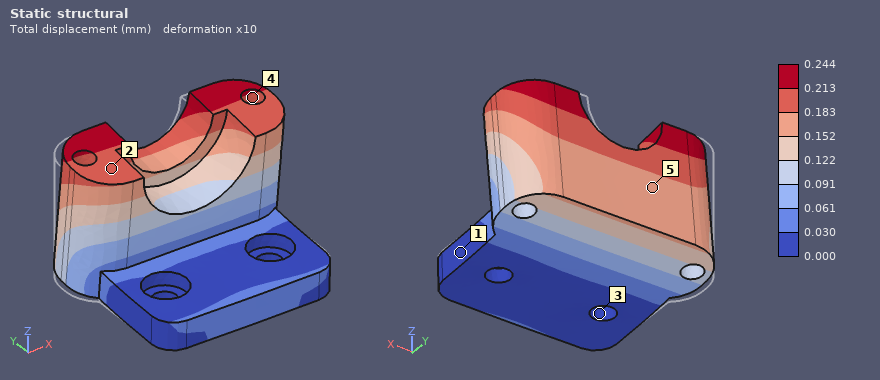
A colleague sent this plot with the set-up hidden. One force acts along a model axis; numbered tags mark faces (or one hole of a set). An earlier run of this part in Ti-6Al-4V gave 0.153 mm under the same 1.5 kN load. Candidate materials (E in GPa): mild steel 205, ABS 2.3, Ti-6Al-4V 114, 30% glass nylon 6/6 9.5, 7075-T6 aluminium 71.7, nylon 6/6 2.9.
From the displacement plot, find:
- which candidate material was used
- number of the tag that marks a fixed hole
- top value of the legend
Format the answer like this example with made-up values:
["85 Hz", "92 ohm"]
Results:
["7075-T6 aluminium", "3", "0.244 mm"]
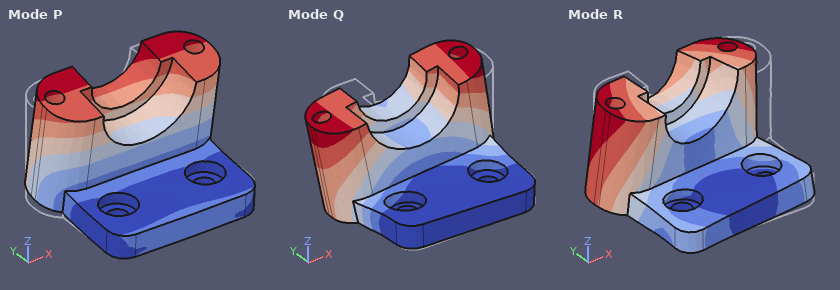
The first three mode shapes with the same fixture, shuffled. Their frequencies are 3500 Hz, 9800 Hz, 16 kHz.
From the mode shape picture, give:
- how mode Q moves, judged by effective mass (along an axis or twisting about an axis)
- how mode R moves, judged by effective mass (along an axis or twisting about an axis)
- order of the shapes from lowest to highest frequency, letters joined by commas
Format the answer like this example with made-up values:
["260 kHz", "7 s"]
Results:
["along X", "along X", "P, Q, R"]
